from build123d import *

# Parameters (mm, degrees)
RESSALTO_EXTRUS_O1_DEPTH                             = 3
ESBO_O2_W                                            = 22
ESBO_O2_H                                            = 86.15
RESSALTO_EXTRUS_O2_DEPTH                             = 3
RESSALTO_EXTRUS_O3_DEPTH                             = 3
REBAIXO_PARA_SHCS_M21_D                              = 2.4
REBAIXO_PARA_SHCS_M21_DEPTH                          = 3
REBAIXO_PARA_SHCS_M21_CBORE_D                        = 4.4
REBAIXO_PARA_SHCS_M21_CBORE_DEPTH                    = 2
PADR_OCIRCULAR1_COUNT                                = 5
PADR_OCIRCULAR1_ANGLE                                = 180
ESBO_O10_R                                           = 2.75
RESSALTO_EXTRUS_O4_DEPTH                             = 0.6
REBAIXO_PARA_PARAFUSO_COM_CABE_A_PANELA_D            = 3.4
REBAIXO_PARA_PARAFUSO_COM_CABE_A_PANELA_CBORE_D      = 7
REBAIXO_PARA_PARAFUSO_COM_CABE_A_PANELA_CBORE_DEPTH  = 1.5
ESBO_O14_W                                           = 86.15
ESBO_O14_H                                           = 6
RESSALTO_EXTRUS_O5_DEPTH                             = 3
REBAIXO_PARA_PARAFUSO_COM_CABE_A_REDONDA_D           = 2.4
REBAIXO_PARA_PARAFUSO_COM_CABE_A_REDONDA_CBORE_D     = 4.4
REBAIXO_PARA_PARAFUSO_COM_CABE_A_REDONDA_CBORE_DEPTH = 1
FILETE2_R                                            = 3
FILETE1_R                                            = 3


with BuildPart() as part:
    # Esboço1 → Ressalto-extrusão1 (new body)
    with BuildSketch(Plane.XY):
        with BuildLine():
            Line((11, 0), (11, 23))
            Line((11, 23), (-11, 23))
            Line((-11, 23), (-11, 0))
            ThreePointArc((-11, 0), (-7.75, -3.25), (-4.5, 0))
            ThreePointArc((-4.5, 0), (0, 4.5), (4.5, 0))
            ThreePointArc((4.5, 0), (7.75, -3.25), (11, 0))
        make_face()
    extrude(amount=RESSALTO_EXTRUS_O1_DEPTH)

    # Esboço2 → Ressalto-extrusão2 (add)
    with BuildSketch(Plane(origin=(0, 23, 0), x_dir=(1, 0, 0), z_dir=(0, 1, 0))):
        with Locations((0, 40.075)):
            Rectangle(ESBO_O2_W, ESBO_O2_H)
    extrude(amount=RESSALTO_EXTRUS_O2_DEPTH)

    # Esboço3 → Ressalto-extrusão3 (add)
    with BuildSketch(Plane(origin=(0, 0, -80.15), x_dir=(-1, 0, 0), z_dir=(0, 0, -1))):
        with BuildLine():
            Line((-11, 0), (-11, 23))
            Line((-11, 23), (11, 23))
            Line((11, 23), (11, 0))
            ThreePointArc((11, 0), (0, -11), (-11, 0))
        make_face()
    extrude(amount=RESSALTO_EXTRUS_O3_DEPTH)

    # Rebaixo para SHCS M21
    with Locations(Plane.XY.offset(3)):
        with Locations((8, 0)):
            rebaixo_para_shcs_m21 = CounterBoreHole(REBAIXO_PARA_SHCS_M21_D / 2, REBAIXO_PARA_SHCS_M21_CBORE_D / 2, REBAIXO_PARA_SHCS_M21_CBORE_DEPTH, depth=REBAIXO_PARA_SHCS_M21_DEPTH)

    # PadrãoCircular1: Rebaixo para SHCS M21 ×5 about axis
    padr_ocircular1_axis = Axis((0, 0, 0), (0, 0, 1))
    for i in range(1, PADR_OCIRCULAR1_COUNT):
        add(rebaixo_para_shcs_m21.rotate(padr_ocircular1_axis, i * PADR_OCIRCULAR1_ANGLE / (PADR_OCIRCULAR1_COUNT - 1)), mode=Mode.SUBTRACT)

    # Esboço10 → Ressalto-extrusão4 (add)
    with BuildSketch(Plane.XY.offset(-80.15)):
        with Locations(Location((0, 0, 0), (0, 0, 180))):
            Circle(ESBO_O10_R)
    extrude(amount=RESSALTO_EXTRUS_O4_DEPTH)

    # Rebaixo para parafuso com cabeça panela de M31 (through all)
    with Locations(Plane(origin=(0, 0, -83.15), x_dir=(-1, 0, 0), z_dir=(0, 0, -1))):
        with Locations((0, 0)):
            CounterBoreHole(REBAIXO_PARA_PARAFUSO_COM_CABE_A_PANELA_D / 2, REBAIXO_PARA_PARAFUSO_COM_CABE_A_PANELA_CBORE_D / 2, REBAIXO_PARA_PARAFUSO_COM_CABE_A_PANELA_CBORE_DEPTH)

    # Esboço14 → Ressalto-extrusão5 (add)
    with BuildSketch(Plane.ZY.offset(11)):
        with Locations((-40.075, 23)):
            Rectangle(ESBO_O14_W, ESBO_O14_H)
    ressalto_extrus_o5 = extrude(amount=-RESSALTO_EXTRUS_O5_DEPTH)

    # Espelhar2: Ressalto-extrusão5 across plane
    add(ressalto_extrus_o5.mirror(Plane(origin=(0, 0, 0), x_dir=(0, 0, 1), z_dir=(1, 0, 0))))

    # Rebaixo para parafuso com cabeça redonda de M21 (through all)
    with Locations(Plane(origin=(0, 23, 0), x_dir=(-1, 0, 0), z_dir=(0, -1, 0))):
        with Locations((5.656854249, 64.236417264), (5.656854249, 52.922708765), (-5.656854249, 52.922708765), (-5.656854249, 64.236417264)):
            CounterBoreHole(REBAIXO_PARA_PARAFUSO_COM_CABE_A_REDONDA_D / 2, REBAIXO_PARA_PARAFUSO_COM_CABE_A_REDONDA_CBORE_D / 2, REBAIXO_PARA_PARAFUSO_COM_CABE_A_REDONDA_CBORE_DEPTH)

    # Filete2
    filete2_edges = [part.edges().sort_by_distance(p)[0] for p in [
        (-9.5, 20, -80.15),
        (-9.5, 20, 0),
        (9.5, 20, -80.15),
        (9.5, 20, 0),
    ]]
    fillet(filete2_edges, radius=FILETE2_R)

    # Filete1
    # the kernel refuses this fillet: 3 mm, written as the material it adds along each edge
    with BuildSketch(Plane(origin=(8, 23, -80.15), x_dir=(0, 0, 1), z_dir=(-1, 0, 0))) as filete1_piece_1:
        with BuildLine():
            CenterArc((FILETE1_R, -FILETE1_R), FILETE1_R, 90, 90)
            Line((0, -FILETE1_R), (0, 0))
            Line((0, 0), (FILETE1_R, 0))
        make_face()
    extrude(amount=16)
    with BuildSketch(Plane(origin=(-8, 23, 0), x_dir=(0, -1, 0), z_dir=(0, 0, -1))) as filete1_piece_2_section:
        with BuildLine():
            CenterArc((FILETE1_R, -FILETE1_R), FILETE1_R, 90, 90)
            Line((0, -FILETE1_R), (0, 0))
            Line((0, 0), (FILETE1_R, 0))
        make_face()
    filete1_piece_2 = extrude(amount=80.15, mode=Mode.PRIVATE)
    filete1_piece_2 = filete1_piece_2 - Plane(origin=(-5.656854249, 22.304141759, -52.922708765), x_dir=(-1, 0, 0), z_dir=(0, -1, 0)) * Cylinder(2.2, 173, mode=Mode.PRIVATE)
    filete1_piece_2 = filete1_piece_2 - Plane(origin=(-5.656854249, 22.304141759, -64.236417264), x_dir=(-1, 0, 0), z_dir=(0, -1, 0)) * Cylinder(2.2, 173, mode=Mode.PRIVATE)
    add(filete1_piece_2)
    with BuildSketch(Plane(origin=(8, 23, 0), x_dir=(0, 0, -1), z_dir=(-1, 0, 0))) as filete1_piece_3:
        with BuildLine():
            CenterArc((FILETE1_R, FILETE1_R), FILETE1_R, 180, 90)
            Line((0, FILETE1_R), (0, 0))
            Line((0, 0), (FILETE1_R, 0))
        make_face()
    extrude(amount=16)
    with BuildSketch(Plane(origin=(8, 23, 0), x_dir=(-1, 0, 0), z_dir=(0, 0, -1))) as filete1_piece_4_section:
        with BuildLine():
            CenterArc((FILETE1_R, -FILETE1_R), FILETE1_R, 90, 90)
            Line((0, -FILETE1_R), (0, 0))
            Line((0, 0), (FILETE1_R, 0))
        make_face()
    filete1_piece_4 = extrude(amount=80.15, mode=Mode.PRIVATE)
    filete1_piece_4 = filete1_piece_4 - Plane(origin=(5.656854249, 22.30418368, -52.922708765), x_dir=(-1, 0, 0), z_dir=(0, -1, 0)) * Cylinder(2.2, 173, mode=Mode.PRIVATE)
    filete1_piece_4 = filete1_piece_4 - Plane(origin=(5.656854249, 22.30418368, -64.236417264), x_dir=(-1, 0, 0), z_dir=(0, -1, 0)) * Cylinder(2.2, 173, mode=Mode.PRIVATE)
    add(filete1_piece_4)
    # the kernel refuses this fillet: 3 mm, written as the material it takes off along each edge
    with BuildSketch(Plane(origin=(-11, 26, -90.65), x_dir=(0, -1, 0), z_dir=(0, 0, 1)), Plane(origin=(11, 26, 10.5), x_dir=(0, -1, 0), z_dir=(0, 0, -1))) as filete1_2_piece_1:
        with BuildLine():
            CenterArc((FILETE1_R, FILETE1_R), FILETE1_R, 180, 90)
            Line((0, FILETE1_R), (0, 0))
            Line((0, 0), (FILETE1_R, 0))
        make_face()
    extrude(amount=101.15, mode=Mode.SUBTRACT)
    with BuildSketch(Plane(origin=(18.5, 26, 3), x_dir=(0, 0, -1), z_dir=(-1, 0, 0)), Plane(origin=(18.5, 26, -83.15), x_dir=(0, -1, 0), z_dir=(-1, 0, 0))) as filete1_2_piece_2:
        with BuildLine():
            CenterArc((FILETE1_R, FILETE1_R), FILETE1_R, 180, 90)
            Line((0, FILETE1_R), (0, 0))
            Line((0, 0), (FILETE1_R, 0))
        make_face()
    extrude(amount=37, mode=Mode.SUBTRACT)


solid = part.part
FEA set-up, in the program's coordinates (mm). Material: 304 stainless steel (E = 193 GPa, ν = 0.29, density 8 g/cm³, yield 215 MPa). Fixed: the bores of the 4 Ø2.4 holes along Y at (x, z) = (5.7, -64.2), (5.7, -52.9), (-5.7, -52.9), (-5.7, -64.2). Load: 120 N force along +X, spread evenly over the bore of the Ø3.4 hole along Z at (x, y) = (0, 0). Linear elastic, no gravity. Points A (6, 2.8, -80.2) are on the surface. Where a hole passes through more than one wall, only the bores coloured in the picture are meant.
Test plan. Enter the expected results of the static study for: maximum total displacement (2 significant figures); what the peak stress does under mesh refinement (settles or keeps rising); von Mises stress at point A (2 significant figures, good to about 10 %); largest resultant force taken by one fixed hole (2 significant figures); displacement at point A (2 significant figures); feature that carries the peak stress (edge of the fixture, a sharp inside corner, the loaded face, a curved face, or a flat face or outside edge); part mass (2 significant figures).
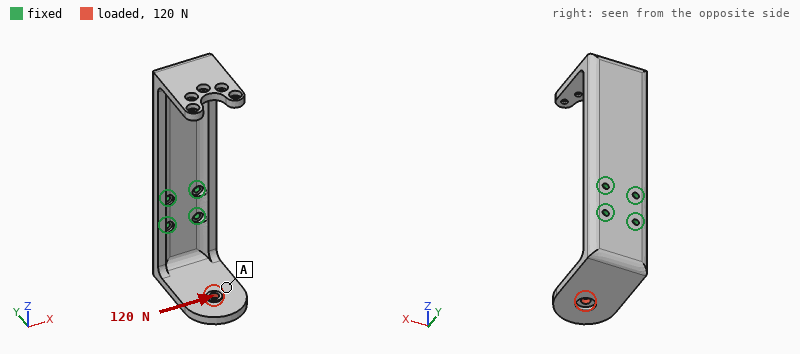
49 µm
keeps rising
7.2 MPa
350 N
32 µm
edge of the fixture
83 g
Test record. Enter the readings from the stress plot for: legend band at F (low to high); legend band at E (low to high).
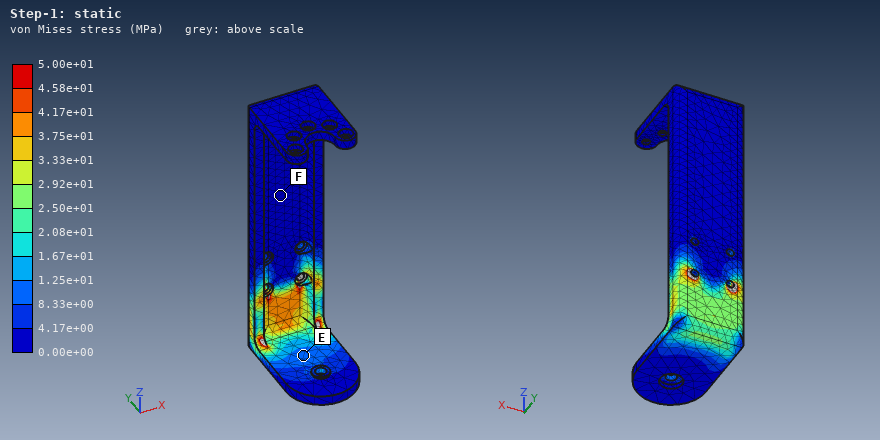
0.00e+00 to 4.17e+00 MPa
8.33e+00 to 1.25e+01 MPa
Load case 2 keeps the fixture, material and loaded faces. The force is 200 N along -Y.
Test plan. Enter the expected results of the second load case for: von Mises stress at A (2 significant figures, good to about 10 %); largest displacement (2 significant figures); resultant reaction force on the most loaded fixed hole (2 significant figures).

7.4 MPa
32 µm
250 N
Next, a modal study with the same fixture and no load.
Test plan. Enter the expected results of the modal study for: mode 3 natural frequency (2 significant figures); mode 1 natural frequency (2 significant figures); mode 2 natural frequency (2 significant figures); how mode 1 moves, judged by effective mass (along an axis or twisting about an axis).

1800 Hz
820 Hz
1800 Hz
along Y
